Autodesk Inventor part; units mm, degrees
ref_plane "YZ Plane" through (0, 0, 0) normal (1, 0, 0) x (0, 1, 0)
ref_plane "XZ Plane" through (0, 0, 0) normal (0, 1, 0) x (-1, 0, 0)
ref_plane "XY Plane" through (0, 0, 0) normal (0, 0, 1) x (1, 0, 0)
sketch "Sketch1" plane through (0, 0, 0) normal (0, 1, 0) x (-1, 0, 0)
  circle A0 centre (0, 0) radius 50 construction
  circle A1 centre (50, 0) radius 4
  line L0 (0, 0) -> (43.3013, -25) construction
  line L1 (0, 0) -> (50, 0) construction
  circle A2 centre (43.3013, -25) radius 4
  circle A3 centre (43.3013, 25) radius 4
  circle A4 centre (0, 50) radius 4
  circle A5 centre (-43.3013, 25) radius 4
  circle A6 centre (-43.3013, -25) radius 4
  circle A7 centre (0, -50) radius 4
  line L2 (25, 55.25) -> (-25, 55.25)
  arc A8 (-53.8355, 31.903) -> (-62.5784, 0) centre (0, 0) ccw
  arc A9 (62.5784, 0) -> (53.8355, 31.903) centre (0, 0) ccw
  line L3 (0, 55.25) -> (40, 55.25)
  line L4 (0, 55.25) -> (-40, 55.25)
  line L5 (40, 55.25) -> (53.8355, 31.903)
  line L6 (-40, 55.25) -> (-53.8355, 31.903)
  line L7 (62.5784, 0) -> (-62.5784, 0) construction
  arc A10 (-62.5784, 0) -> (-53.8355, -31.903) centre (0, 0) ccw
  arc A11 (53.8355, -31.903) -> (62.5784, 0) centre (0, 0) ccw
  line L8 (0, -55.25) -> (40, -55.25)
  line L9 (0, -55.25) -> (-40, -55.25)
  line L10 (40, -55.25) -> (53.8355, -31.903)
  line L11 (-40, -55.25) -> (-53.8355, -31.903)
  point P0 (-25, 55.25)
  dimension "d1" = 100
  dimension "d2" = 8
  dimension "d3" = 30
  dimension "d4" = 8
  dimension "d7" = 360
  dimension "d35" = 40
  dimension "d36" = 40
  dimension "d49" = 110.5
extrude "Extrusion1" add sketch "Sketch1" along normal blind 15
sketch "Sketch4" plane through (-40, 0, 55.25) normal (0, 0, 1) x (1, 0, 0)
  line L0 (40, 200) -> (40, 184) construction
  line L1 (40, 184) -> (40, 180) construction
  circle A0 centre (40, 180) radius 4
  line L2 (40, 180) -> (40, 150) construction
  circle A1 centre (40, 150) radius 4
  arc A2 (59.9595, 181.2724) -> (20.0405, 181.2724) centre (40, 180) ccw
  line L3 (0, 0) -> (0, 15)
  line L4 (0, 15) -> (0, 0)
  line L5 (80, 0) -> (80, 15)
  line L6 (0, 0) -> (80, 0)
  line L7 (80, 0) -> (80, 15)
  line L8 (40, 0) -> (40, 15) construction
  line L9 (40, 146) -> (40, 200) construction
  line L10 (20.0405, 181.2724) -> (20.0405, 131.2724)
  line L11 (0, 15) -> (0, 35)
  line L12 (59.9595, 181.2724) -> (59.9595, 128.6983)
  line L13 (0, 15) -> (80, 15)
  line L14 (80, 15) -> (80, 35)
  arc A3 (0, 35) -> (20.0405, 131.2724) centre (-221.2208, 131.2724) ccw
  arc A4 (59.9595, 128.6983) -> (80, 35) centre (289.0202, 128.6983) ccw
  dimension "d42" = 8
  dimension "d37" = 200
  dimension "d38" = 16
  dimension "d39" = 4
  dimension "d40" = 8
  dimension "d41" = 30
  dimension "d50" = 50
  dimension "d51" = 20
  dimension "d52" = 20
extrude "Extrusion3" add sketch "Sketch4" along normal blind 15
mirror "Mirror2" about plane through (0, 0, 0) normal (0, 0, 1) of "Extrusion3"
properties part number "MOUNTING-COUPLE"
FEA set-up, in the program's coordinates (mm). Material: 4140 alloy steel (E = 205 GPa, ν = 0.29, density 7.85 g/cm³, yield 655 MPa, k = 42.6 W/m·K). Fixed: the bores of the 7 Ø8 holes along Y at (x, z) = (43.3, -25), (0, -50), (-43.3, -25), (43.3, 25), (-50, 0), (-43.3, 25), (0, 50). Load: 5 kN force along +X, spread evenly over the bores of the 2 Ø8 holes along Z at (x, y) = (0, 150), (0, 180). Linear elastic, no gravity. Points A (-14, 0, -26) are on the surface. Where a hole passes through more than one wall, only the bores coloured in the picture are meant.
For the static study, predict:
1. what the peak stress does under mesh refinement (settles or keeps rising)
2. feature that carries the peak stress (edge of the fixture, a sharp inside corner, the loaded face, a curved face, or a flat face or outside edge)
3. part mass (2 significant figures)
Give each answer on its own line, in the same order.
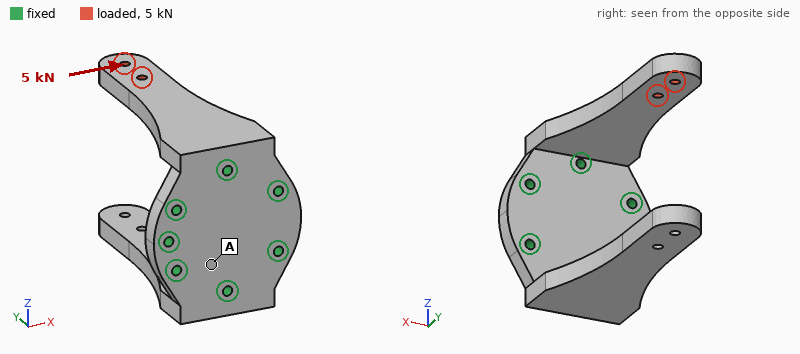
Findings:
keeps rising
edge of the fixture
3.8 kg
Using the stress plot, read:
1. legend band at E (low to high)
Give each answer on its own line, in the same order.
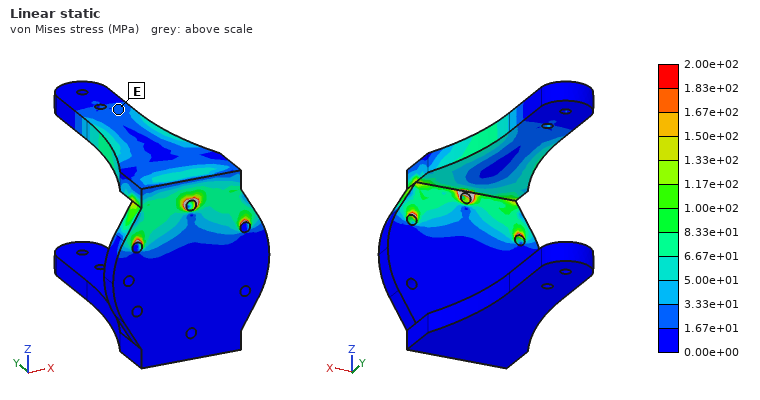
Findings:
1.67e+01 to 3.33e+01 MPa
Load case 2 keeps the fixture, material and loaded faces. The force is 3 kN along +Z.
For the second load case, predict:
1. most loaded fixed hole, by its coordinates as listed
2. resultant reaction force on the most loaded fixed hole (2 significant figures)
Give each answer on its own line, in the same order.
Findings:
(0, 50)
7.8 kN
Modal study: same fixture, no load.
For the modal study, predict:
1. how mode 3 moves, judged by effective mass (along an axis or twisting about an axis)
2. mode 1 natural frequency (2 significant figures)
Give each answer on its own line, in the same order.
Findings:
along X
410 Hz
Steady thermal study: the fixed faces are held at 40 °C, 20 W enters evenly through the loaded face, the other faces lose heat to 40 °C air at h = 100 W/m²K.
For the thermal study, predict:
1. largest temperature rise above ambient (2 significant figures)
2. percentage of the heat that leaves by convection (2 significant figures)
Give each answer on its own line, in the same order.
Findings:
23 K
95 %
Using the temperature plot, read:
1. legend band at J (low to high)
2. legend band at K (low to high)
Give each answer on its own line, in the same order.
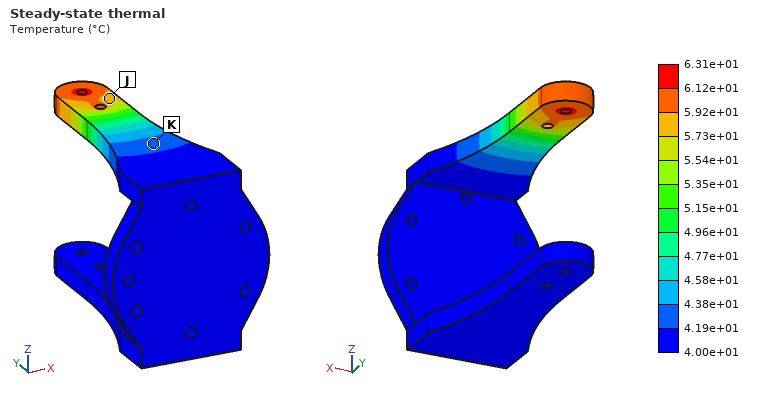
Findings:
5.73e+01 to 5.92e+01 °C
4.19e+01 to 4.38e+01 °C
